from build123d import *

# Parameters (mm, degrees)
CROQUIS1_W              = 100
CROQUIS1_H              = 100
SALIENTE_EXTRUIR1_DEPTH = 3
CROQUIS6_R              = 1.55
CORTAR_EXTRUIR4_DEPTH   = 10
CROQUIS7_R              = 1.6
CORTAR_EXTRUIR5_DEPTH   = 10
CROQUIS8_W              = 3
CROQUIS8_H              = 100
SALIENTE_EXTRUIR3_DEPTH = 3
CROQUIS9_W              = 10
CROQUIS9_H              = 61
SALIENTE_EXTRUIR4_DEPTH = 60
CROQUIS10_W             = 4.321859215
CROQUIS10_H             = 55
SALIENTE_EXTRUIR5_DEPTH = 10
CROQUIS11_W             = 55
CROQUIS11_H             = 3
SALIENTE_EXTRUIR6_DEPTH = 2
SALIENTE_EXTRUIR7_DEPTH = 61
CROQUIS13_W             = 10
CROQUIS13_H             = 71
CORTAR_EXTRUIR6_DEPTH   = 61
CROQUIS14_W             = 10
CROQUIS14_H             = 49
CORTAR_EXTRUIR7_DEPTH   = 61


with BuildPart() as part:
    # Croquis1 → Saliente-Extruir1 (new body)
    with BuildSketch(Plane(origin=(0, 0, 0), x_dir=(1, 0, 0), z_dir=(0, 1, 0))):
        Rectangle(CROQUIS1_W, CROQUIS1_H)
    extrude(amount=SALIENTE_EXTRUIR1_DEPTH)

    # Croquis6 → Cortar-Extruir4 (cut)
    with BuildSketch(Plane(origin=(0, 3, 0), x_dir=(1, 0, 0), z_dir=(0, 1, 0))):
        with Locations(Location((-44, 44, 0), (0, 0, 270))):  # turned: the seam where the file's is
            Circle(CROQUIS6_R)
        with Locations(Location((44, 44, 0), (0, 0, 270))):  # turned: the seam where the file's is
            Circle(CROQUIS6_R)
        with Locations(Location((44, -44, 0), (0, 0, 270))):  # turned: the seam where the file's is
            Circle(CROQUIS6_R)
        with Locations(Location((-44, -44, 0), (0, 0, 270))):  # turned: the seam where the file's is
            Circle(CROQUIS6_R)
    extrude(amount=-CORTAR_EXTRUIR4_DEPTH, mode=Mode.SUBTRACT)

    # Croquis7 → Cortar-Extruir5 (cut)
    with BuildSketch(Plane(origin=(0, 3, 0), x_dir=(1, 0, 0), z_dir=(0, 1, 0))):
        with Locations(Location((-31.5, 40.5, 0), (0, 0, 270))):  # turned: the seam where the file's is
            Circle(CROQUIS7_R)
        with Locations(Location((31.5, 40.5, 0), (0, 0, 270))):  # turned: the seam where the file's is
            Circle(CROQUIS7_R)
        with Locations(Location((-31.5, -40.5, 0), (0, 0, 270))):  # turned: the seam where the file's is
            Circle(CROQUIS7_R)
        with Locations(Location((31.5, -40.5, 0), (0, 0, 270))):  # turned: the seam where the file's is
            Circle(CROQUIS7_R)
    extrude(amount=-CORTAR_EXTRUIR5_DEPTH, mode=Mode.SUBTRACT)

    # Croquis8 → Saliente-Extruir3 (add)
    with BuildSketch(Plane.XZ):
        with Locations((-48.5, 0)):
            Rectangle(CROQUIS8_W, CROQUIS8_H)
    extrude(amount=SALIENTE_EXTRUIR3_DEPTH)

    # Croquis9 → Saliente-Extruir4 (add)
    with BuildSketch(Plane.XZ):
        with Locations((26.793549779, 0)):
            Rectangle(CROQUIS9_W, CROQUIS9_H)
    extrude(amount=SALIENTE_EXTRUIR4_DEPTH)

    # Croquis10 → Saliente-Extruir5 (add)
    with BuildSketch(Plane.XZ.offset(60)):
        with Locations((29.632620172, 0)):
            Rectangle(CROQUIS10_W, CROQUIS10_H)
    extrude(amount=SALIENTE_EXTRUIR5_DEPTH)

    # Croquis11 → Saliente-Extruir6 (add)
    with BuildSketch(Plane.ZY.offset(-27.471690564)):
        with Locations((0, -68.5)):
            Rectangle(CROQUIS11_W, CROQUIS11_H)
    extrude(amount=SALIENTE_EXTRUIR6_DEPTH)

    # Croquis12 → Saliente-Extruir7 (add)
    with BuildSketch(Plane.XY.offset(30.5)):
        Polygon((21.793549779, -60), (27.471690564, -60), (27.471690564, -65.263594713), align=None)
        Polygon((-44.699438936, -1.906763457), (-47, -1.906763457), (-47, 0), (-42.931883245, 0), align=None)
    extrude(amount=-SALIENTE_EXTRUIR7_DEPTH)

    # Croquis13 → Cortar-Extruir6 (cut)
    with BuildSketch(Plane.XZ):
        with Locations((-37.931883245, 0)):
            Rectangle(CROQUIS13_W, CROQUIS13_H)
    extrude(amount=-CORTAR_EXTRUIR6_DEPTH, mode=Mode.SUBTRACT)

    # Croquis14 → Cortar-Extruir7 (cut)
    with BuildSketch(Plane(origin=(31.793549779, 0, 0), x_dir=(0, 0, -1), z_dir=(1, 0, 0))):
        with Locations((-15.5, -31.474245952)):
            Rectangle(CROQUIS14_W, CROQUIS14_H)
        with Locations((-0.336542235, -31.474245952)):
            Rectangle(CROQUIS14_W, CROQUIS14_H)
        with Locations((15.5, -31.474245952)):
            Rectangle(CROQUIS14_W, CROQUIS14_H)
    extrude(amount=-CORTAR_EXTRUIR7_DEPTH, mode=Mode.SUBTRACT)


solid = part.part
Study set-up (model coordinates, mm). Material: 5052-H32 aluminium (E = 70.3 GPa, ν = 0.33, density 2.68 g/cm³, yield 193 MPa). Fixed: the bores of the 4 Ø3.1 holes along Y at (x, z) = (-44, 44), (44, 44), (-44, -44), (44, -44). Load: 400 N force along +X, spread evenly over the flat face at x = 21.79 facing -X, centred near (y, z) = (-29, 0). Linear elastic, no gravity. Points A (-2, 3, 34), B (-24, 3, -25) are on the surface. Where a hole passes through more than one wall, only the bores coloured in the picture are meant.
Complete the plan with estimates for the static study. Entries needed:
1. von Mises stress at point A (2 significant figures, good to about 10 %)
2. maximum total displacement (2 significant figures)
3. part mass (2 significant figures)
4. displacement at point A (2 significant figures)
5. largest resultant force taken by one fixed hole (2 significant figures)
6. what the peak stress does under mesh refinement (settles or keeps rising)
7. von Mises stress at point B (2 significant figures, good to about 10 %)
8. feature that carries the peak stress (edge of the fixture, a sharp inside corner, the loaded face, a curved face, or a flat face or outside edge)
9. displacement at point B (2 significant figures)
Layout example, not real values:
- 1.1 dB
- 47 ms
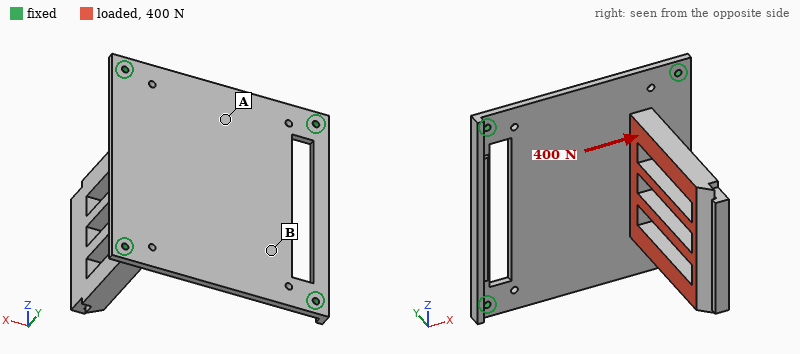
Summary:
- 19 MPa
- 0.59 mm
- 150 g
- 0.13 mm
- 160 N
- keeps rising
- 8.8 MPa
- edge of the fixture
- 0.095 mm
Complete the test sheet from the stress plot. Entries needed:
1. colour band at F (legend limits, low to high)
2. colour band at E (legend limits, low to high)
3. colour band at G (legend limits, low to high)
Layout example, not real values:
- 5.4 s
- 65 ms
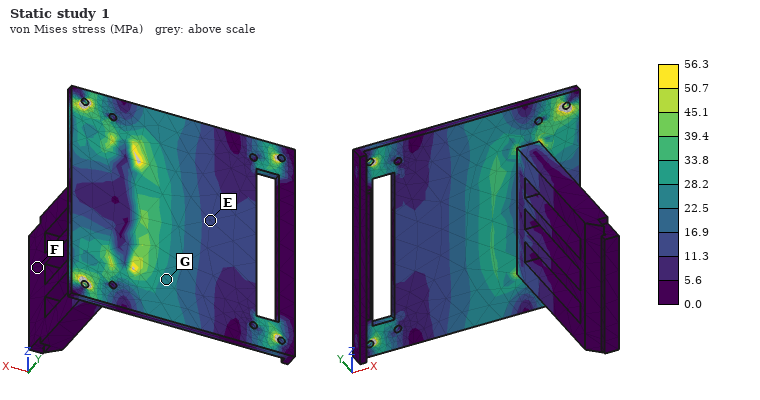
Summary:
- 0.0 to 5.6 MPa
- 11.3 to 16.9 MPa
- 22.5 to 28.2 MPa
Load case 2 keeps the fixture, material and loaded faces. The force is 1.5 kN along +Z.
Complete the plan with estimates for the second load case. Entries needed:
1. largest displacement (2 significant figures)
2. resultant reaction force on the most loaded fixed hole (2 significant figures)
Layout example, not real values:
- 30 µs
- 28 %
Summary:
- 0.39 mm
- 890 N
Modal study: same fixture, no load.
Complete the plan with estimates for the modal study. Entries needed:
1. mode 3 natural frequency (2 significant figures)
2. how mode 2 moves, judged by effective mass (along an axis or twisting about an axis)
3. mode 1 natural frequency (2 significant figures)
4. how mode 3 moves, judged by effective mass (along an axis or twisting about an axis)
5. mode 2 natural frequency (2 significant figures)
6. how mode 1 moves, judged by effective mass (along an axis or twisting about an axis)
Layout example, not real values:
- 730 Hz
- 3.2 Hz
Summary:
- 1300 Hz
- along Z
- 530 Hz
- along Y
- 1200 Hz
- along X
